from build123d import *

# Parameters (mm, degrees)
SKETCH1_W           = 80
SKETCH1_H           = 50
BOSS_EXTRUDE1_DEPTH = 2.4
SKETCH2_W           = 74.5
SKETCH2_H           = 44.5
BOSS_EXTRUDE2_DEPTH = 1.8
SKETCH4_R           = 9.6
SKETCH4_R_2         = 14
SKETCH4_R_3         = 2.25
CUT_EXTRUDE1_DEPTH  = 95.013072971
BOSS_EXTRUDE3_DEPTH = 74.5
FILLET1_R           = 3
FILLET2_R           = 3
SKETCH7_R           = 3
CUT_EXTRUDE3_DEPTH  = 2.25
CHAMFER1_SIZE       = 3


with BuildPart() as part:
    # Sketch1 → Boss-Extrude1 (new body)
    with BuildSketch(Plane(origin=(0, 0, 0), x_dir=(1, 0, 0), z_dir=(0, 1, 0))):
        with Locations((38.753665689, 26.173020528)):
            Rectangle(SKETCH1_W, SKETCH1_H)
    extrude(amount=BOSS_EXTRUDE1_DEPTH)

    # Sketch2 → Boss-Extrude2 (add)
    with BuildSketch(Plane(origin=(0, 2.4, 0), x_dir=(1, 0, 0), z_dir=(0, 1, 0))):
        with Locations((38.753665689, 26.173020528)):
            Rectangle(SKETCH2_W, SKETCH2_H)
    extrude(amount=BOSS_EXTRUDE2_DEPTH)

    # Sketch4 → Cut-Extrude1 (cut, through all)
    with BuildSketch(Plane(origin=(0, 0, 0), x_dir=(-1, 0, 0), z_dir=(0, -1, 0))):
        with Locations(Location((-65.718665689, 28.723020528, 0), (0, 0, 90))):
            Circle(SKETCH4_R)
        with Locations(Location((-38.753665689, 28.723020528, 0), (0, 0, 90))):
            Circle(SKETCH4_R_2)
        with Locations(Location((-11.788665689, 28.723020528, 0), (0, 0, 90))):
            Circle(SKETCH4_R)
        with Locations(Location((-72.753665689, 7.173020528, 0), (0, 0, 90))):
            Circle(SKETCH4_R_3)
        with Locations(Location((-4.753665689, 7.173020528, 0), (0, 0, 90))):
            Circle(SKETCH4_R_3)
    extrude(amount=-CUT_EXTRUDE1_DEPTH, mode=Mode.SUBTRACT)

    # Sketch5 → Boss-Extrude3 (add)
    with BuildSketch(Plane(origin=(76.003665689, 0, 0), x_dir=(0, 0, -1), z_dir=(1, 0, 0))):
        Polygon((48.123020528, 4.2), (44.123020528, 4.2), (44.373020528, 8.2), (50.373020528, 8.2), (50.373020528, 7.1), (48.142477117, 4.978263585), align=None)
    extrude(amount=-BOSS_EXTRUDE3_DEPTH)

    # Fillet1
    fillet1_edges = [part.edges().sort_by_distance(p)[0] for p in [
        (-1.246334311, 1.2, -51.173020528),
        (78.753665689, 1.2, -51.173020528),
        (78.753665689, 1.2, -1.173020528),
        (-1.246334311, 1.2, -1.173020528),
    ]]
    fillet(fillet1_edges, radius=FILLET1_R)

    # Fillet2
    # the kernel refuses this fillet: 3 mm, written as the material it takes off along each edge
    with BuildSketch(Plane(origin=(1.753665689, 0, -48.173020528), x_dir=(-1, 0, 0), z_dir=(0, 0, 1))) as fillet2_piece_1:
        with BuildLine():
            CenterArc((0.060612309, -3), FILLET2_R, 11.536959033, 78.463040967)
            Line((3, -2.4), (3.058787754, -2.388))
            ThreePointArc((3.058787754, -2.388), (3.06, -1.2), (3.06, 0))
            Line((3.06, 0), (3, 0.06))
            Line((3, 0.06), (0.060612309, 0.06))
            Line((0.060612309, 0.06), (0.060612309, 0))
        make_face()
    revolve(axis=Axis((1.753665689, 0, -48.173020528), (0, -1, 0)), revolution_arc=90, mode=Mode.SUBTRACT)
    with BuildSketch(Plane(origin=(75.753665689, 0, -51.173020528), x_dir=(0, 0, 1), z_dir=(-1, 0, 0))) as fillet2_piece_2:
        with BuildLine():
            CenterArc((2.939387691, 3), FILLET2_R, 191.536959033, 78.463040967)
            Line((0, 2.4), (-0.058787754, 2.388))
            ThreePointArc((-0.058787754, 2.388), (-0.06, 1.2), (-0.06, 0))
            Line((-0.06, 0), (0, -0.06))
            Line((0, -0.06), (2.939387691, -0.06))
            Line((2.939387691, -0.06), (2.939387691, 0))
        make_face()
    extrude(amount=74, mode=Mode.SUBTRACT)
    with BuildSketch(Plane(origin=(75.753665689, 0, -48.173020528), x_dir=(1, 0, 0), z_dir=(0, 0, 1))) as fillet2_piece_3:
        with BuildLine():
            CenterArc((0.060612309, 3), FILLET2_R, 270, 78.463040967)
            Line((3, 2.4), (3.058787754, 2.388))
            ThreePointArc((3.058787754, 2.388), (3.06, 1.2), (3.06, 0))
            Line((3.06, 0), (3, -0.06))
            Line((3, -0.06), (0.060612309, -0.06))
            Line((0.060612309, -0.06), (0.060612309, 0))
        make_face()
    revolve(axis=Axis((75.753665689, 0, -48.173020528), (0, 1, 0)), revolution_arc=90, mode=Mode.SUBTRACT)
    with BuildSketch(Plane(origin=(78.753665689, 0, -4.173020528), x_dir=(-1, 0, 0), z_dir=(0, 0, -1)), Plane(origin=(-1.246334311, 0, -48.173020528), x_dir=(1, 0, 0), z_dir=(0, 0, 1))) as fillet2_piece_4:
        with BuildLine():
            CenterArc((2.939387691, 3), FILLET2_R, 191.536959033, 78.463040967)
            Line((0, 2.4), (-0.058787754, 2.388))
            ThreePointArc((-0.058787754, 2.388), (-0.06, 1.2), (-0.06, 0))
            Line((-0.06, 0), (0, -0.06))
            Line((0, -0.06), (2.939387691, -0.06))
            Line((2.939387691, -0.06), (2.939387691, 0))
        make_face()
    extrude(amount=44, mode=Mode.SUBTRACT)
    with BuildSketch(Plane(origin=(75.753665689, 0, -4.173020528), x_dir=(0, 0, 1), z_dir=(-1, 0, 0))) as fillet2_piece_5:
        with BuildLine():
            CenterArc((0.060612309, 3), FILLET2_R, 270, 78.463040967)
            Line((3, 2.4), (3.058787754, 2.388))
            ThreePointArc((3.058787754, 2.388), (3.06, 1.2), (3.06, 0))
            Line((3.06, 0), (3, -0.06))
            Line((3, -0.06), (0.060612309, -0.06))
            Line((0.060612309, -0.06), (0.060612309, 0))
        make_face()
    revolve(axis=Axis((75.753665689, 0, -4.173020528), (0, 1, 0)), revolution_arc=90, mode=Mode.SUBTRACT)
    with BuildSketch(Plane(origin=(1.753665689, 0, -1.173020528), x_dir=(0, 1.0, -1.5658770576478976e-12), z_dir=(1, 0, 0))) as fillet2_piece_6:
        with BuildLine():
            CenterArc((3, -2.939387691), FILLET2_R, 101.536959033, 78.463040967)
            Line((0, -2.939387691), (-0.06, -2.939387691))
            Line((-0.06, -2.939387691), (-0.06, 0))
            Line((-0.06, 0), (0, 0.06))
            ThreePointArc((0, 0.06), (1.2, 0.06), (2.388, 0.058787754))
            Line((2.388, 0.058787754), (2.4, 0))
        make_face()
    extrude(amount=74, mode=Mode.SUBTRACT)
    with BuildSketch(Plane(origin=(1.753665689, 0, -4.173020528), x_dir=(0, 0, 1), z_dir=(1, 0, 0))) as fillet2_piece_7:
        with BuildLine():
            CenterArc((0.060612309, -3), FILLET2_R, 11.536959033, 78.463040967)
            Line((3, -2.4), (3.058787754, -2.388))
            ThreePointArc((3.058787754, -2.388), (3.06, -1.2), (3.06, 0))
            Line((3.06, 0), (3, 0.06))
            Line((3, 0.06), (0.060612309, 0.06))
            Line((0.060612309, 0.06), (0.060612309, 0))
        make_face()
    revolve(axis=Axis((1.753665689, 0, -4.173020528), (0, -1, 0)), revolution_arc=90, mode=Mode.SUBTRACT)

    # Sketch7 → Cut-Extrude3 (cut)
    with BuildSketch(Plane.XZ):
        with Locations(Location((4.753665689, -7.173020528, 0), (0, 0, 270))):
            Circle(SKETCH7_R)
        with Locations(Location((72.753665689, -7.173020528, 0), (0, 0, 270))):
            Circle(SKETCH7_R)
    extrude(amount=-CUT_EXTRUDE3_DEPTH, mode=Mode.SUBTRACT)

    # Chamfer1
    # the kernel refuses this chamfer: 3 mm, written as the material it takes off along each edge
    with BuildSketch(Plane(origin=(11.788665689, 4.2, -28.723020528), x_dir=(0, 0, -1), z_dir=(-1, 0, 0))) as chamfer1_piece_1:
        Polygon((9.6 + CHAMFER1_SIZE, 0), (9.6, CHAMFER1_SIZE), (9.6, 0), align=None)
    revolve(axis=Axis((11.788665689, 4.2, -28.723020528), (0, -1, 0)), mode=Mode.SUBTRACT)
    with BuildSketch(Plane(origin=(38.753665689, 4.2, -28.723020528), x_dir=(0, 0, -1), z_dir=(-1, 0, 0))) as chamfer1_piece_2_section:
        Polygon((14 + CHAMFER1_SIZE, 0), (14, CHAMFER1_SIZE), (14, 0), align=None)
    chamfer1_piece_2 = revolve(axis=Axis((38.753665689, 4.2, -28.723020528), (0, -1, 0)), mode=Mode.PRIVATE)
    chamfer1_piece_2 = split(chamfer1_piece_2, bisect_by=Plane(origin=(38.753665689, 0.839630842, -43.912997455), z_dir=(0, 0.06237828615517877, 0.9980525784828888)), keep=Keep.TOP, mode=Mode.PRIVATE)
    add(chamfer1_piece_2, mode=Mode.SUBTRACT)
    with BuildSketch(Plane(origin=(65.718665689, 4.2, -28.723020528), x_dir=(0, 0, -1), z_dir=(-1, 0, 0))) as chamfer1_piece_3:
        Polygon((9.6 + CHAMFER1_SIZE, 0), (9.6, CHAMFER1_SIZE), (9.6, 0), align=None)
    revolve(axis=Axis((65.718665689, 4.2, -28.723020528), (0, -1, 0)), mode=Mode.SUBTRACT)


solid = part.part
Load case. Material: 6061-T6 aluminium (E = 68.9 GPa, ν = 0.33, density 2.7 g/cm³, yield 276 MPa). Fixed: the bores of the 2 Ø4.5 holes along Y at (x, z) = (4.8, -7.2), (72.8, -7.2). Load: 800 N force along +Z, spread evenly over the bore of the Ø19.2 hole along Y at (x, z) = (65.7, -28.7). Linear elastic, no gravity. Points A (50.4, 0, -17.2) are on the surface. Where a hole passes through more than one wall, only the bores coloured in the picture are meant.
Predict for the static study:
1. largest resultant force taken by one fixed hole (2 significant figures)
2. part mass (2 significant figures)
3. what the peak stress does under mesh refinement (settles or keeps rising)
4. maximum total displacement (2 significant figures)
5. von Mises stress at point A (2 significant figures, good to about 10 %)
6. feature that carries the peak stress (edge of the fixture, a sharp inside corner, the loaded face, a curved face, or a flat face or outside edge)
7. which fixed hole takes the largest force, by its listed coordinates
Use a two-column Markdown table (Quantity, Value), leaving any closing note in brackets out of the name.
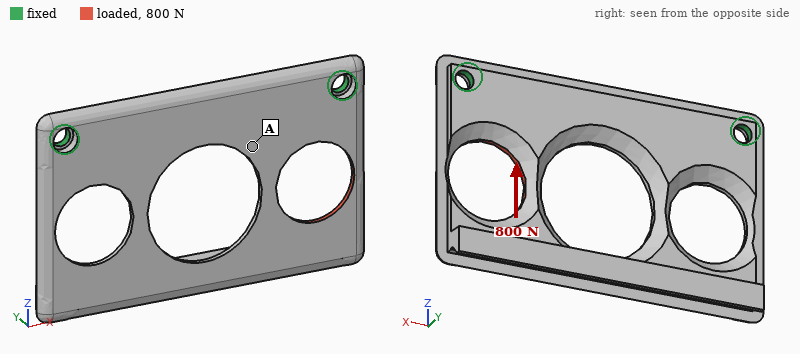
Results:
| Quantity | Value |
|---|---|
| largest resultant force taken by one fixed hole | 720 N |
| part mass | 28 g |
| what the peak stress does under mesh refinement | keeps rising |
| maximum total displacement | 0.20 mm |
| von Mises stress at point A | 13 MPa |
| feature that carries the peak stress | edge of the fixture |
| which fixed hole takes the largest force, by its listed coordinates | (72.8, -7.2) |
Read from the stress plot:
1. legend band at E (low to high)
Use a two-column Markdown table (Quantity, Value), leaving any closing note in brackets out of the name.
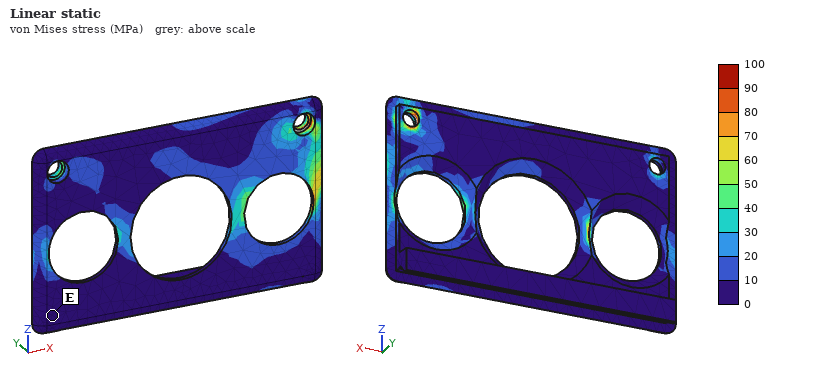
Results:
| Quantity | Value |
|---|---|
| legend band at E | 0 to 10 MPa |
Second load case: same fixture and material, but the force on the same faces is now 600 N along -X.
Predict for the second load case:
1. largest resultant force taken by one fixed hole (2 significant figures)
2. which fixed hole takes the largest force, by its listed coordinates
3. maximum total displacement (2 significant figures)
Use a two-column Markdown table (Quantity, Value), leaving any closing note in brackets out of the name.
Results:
| Quantity | Value |
|---|---|
| largest resultant force taken by one fixed hole | 390 N |
| which fixed hole takes the largest force, by its listed coordinates | (72.8, -7.2) |
| maximum total displacement | 39 µm |
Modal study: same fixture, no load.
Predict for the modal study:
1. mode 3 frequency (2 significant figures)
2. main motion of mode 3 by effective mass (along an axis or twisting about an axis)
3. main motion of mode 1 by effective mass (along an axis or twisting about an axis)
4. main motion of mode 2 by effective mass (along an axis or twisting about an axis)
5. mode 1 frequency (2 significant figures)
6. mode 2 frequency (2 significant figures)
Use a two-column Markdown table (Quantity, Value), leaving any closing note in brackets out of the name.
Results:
| Quantity | Value |
|---|---|
| mode 3 frequency | 3800 Hz |
| main motion of mode 3 by effective mass | along Y |
| main motion of mode 1 by effective mass | along Y |
| main motion of mode 2 by effective mass | twisting about Z |
| mode 1 frequency | 600 Hz |
| mode 2 frequency | 1700 Hz |
